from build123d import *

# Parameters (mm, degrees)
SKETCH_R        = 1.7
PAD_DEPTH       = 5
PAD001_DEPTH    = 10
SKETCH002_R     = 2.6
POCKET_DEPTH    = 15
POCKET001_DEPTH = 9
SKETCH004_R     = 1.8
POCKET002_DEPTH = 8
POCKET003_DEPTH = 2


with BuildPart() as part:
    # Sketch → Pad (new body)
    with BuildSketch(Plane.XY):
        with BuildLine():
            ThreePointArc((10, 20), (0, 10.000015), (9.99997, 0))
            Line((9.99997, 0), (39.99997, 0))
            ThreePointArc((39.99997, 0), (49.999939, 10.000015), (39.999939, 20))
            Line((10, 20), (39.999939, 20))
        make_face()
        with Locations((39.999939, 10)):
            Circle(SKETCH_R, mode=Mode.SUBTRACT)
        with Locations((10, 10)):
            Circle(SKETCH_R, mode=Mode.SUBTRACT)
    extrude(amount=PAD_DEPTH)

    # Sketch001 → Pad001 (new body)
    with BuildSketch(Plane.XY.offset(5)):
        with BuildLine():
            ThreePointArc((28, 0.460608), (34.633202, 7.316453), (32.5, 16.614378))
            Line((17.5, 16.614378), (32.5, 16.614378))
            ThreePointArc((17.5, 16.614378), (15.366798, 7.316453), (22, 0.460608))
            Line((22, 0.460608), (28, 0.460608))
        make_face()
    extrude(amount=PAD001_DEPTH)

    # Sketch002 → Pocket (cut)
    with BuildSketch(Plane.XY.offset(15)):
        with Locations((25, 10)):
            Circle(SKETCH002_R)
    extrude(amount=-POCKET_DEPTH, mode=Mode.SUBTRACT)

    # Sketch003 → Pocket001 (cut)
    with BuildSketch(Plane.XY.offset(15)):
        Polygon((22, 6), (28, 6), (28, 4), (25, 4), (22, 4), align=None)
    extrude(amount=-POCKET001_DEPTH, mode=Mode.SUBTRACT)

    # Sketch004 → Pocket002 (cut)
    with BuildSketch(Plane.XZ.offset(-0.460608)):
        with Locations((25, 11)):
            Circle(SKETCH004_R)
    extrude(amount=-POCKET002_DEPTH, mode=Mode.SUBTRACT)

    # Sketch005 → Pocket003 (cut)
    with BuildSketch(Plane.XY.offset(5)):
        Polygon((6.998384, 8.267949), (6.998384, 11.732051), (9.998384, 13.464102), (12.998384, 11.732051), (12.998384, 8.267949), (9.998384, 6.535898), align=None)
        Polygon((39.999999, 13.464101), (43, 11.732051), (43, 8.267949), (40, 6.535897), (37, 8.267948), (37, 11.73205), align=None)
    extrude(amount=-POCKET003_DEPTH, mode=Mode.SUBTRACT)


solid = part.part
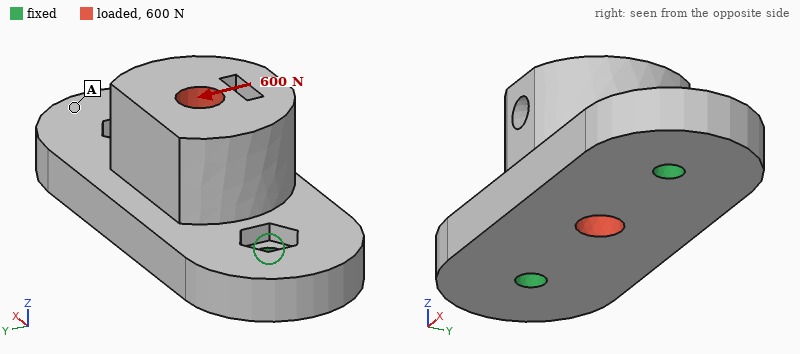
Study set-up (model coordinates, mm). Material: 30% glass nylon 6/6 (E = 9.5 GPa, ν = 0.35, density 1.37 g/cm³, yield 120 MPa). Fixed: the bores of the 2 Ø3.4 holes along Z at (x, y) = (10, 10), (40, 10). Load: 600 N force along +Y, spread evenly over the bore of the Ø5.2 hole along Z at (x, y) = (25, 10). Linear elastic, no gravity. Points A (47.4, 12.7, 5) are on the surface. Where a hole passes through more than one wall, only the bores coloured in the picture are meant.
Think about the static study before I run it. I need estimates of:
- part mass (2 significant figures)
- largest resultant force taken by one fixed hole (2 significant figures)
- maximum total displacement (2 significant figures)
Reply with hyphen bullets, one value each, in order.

- 9.2 g
- 300 N
- 0.17 mm
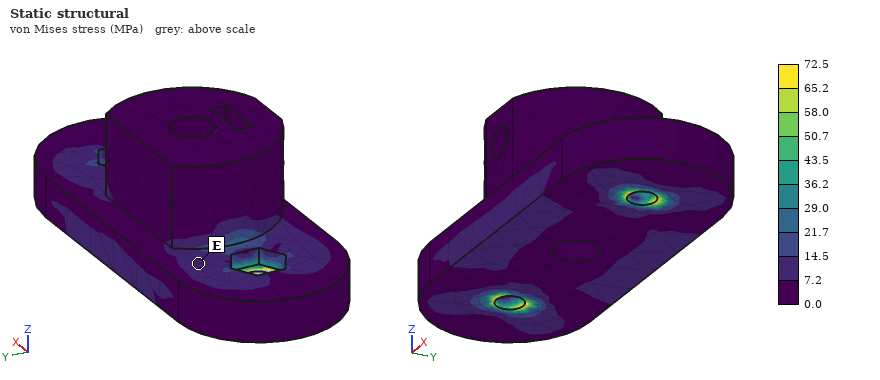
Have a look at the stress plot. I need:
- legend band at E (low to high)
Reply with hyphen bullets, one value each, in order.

- 7.2 to 14.5 MPa
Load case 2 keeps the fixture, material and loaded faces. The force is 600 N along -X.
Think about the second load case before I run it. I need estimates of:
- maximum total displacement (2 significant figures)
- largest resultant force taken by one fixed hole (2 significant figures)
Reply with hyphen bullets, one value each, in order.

- 17 µm
- 320 N
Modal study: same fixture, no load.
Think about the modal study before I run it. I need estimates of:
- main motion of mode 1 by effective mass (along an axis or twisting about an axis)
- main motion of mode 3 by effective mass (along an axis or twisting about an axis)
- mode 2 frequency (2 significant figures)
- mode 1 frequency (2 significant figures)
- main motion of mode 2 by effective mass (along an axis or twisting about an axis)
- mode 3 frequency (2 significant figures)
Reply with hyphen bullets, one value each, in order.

- along Y
- along X
- 9300 Hz
- 4400 Hz
- along Z
- 14 kHz
